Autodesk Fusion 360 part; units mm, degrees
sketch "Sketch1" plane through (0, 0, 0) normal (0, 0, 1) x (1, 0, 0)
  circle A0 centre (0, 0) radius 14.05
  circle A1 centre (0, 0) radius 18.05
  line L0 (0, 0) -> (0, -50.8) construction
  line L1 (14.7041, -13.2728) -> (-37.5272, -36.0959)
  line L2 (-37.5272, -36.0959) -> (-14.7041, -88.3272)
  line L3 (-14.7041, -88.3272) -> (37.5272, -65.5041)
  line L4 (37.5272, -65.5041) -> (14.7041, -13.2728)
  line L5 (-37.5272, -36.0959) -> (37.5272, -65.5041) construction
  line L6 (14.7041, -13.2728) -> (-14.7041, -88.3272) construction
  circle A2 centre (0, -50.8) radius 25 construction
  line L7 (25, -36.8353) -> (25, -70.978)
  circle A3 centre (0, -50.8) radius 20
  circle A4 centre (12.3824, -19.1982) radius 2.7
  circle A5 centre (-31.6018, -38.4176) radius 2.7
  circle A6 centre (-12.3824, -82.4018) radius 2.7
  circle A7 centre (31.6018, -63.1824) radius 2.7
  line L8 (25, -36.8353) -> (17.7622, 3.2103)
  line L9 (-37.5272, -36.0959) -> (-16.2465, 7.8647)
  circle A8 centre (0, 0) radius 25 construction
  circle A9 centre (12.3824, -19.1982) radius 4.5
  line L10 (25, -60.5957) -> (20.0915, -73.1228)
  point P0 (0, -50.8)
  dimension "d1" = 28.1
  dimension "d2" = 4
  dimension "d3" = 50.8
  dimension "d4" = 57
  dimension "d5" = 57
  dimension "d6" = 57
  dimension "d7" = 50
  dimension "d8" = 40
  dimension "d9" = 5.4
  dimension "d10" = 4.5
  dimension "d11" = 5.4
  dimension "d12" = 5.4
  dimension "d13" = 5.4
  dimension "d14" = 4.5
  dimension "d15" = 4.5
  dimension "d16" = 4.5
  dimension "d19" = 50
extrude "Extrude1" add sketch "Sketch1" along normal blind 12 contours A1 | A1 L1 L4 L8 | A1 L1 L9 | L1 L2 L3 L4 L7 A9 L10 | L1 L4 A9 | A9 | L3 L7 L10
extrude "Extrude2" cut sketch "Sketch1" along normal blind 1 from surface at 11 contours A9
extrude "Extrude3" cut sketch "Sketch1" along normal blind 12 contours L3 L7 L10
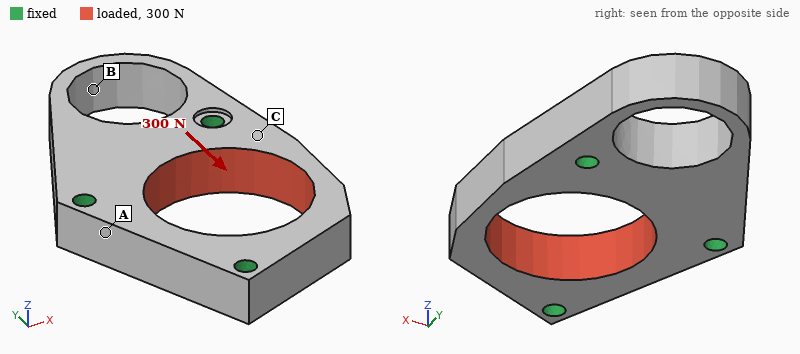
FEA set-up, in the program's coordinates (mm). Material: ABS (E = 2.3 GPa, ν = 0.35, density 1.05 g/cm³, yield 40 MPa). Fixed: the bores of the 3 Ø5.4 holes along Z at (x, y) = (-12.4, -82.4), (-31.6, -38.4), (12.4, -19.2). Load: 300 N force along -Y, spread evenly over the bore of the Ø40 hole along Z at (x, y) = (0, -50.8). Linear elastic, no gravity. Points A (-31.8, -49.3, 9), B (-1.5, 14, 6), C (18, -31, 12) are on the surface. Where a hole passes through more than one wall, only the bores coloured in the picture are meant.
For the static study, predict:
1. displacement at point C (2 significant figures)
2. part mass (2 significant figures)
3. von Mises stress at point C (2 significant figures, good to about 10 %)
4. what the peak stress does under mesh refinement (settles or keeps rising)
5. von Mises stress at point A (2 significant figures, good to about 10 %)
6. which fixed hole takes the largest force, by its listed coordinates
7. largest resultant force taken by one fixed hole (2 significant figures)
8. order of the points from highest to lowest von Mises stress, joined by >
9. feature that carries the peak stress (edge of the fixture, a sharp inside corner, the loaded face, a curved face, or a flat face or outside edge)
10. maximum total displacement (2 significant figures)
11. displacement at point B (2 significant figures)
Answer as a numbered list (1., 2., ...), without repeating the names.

1. 5.8 µm
2. 34 g
3. 0.74 MPa
4. keeps rising
5. 0.40 MPa
6. (12.4, -19.2)
7. 140 N
8. C > A > B
9. edge of the fixture
10. 22 µm
11. 3.6 µm
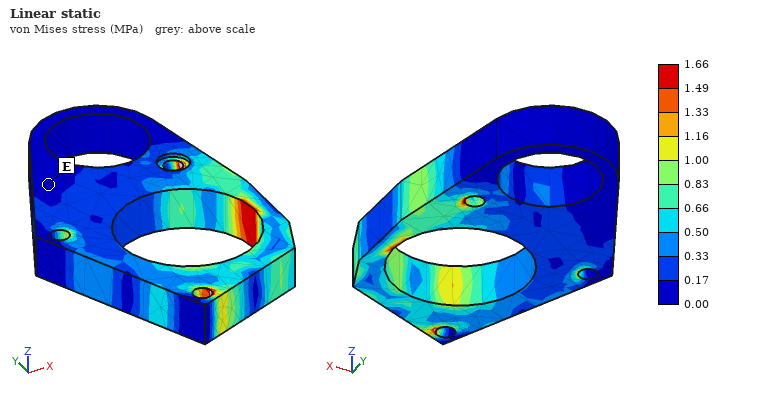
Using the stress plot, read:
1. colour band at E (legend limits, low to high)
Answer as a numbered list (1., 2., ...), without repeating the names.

1. 0.00 to 0.17 MPa
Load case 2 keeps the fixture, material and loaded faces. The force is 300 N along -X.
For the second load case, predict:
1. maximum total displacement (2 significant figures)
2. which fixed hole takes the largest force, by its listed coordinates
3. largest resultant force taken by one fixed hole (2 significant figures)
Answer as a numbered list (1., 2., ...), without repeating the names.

1. 26 µm
2. (-12.4, -82.4)
3. 130 N
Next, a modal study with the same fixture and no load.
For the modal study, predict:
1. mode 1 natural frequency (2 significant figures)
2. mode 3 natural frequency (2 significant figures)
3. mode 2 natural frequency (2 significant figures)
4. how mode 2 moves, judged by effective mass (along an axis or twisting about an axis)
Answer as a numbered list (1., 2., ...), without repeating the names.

1. 1800 Hz
2. 2800 Hz
3. 2400 Hz
4. along Z
